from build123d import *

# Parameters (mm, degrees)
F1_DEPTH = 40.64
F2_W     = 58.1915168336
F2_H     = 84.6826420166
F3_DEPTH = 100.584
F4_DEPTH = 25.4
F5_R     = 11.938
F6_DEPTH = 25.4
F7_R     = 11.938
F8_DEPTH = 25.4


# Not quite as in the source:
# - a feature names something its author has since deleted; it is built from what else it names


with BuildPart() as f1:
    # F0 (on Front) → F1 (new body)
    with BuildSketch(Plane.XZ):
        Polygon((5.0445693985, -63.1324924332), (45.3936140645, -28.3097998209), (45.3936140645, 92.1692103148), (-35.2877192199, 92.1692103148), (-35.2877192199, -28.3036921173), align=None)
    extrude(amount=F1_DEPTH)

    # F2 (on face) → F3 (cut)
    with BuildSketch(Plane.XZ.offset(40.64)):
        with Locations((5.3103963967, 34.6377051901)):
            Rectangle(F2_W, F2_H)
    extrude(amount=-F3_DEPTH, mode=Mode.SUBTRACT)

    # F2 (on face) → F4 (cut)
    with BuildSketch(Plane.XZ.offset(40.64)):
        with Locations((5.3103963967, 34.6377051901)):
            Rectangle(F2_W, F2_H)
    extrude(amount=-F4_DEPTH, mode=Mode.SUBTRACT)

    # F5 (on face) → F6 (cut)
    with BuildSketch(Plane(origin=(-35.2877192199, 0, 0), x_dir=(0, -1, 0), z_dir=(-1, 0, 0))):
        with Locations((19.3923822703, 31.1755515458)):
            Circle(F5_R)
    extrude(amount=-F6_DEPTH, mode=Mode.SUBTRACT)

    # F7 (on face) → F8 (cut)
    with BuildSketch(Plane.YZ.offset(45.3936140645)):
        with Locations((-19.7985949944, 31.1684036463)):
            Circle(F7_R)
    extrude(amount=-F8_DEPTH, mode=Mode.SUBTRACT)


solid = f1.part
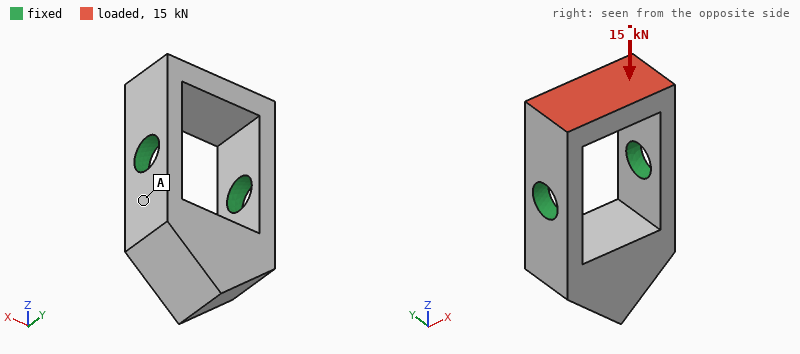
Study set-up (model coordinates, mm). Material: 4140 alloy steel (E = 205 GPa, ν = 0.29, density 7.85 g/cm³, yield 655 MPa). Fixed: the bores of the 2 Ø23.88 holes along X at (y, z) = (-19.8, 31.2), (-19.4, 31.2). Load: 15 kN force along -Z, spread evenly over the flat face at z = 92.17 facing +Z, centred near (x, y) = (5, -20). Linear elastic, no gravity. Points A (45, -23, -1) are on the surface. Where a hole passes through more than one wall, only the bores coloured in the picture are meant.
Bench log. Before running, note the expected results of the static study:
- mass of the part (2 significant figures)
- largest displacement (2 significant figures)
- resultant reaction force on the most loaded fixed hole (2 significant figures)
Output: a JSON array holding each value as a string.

["1.9 kg", "17 µm", "7.7 kN"]
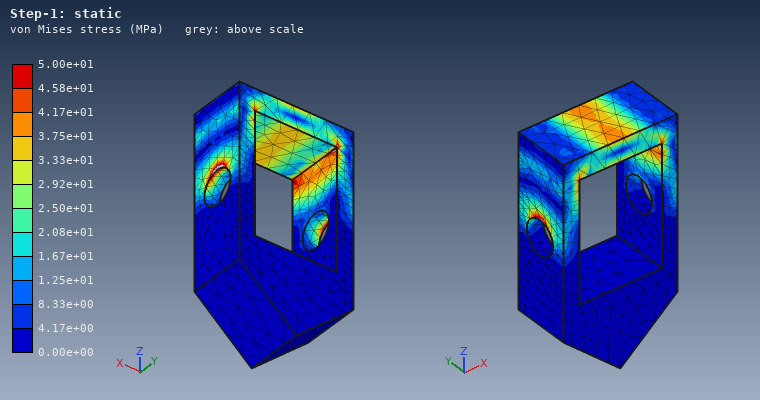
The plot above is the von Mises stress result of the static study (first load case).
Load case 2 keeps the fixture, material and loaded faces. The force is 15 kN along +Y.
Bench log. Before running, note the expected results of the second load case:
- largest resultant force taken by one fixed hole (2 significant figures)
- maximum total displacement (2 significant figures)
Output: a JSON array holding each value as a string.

["7.6 kN", "64 µm"]
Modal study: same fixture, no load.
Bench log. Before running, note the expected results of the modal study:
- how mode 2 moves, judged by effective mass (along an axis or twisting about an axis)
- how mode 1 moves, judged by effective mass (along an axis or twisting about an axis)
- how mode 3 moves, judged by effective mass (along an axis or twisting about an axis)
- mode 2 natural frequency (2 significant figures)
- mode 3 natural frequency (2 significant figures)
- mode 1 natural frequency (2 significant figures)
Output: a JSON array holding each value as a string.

["along X", "along Y", "along X", "3100 Hz", "3500 Hz", "2600 Hz"]
